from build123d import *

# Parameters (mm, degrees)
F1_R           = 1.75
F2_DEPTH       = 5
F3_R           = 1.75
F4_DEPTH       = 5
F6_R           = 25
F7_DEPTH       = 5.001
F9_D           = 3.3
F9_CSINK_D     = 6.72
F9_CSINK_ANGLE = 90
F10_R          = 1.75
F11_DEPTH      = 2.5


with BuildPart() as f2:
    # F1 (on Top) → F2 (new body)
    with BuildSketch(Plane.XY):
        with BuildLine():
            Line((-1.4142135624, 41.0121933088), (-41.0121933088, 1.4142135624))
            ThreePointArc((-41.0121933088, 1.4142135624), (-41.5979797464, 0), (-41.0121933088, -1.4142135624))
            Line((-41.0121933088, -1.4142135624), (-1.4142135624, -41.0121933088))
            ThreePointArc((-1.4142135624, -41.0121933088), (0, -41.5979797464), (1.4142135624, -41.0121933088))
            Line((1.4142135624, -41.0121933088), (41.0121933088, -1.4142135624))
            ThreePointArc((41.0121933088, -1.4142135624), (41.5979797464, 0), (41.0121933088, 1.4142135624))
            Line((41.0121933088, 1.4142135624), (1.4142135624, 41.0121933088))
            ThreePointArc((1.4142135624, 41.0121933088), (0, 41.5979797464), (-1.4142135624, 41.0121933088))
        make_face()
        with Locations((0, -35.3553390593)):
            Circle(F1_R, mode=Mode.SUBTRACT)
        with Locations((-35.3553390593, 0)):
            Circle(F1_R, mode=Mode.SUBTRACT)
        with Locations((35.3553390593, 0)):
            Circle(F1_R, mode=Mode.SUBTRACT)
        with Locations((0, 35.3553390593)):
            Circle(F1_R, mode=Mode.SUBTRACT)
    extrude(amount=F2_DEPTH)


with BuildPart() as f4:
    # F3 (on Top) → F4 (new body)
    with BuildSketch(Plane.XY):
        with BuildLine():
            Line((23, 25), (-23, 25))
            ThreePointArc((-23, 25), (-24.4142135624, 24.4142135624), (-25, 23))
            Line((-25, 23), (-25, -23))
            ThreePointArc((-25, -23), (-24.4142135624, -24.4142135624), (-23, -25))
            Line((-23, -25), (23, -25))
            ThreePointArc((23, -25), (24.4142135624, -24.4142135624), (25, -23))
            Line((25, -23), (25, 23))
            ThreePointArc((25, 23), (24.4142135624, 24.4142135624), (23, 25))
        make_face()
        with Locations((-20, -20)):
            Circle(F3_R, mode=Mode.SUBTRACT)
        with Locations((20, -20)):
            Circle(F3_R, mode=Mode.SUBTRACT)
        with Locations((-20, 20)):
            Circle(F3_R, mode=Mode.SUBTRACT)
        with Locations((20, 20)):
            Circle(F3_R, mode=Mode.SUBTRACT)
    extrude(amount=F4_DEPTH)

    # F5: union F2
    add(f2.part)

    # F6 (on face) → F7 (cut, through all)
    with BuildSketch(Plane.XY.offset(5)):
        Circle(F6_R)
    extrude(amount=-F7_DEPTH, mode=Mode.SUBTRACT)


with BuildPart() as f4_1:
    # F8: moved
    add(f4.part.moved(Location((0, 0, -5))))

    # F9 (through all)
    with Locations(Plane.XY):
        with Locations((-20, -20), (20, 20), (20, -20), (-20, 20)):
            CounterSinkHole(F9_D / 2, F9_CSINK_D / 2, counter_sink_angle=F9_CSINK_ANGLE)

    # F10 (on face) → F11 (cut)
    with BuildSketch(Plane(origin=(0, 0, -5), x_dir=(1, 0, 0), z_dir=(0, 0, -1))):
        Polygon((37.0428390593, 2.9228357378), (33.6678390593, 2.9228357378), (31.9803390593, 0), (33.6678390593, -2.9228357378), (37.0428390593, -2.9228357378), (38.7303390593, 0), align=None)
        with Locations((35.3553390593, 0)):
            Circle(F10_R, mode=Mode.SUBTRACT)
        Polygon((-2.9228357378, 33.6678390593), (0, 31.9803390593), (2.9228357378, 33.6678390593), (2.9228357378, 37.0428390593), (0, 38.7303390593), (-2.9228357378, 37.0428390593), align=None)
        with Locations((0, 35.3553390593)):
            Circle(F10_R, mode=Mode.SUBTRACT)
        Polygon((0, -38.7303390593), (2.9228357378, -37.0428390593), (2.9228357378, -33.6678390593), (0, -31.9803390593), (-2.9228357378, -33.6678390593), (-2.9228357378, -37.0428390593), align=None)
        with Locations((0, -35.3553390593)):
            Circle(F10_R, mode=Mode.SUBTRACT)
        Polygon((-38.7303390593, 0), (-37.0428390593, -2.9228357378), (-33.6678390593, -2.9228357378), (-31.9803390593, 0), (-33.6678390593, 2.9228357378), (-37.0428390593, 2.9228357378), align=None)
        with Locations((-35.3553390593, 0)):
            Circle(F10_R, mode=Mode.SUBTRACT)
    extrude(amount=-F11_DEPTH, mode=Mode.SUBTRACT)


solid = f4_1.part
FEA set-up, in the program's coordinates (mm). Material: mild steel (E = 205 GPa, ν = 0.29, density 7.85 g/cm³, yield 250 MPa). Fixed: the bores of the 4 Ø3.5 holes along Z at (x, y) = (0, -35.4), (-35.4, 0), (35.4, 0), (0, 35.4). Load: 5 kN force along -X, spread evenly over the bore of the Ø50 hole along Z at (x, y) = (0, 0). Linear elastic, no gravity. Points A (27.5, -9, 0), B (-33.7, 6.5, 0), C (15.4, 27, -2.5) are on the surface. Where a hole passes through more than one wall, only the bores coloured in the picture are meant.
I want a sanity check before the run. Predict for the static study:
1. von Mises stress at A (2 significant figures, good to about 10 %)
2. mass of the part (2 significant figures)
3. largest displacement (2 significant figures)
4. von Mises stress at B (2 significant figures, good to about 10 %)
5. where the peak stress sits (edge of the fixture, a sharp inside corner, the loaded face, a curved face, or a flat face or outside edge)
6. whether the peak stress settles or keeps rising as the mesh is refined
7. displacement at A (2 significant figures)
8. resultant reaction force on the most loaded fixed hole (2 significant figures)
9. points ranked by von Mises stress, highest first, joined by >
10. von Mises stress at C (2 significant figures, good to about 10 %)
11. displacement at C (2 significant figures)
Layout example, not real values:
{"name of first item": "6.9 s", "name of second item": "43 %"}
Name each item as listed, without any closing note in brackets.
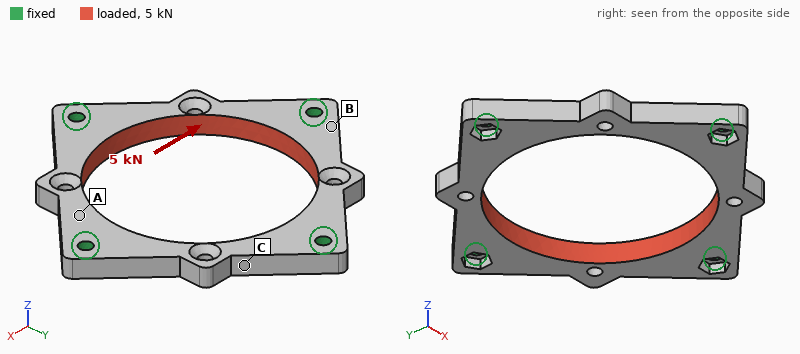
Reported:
{"von Mises stress at A": "20 MPa", "mass of the part": "63 g", "largest displacement": "12 µm", "von Mises stress at B": "34 MPa", "where the peak stress sits": "edge of the fixture", "whether the peak stress settles or keeps rising as the mesh is refined": "keeps rising", "displacement at A": "2.6 µm", "resultant reaction force on the most loaded fixed hole": "1.4 kN", "points ranked by von Mises stress, highest first, joined by >": "C > B > A", "von Mises stress at C": "61 MPa", "displacement at C": "11 µm"}
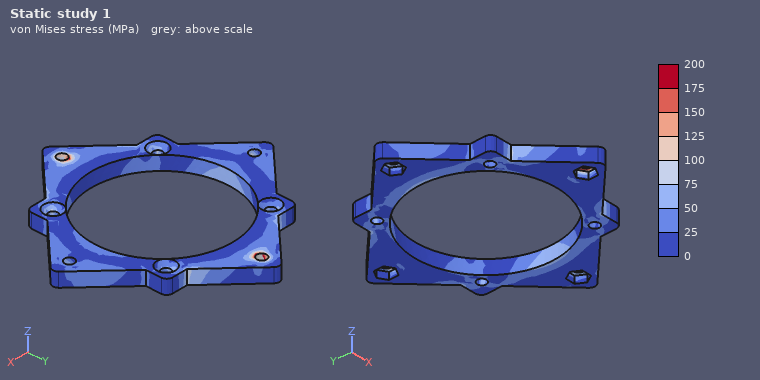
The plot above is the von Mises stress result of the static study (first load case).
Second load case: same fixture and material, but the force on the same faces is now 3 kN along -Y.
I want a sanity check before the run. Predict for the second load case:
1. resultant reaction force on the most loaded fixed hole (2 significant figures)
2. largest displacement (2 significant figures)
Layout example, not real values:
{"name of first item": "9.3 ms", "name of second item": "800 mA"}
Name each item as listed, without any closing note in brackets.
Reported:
{"resultant reaction force on the most loaded fixed hole": "860 N", "largest displacement": "7.0 µm"}
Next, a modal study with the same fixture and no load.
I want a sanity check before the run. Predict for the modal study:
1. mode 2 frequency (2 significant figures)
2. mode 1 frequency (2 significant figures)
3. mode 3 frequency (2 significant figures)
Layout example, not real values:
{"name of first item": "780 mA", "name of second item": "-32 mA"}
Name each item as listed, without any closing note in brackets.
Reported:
{"mode 2 frequency": "8700 Hz", "mode 1 frequency": "7600 Hz", "mode 3 frequency": "8700 Hz"}
